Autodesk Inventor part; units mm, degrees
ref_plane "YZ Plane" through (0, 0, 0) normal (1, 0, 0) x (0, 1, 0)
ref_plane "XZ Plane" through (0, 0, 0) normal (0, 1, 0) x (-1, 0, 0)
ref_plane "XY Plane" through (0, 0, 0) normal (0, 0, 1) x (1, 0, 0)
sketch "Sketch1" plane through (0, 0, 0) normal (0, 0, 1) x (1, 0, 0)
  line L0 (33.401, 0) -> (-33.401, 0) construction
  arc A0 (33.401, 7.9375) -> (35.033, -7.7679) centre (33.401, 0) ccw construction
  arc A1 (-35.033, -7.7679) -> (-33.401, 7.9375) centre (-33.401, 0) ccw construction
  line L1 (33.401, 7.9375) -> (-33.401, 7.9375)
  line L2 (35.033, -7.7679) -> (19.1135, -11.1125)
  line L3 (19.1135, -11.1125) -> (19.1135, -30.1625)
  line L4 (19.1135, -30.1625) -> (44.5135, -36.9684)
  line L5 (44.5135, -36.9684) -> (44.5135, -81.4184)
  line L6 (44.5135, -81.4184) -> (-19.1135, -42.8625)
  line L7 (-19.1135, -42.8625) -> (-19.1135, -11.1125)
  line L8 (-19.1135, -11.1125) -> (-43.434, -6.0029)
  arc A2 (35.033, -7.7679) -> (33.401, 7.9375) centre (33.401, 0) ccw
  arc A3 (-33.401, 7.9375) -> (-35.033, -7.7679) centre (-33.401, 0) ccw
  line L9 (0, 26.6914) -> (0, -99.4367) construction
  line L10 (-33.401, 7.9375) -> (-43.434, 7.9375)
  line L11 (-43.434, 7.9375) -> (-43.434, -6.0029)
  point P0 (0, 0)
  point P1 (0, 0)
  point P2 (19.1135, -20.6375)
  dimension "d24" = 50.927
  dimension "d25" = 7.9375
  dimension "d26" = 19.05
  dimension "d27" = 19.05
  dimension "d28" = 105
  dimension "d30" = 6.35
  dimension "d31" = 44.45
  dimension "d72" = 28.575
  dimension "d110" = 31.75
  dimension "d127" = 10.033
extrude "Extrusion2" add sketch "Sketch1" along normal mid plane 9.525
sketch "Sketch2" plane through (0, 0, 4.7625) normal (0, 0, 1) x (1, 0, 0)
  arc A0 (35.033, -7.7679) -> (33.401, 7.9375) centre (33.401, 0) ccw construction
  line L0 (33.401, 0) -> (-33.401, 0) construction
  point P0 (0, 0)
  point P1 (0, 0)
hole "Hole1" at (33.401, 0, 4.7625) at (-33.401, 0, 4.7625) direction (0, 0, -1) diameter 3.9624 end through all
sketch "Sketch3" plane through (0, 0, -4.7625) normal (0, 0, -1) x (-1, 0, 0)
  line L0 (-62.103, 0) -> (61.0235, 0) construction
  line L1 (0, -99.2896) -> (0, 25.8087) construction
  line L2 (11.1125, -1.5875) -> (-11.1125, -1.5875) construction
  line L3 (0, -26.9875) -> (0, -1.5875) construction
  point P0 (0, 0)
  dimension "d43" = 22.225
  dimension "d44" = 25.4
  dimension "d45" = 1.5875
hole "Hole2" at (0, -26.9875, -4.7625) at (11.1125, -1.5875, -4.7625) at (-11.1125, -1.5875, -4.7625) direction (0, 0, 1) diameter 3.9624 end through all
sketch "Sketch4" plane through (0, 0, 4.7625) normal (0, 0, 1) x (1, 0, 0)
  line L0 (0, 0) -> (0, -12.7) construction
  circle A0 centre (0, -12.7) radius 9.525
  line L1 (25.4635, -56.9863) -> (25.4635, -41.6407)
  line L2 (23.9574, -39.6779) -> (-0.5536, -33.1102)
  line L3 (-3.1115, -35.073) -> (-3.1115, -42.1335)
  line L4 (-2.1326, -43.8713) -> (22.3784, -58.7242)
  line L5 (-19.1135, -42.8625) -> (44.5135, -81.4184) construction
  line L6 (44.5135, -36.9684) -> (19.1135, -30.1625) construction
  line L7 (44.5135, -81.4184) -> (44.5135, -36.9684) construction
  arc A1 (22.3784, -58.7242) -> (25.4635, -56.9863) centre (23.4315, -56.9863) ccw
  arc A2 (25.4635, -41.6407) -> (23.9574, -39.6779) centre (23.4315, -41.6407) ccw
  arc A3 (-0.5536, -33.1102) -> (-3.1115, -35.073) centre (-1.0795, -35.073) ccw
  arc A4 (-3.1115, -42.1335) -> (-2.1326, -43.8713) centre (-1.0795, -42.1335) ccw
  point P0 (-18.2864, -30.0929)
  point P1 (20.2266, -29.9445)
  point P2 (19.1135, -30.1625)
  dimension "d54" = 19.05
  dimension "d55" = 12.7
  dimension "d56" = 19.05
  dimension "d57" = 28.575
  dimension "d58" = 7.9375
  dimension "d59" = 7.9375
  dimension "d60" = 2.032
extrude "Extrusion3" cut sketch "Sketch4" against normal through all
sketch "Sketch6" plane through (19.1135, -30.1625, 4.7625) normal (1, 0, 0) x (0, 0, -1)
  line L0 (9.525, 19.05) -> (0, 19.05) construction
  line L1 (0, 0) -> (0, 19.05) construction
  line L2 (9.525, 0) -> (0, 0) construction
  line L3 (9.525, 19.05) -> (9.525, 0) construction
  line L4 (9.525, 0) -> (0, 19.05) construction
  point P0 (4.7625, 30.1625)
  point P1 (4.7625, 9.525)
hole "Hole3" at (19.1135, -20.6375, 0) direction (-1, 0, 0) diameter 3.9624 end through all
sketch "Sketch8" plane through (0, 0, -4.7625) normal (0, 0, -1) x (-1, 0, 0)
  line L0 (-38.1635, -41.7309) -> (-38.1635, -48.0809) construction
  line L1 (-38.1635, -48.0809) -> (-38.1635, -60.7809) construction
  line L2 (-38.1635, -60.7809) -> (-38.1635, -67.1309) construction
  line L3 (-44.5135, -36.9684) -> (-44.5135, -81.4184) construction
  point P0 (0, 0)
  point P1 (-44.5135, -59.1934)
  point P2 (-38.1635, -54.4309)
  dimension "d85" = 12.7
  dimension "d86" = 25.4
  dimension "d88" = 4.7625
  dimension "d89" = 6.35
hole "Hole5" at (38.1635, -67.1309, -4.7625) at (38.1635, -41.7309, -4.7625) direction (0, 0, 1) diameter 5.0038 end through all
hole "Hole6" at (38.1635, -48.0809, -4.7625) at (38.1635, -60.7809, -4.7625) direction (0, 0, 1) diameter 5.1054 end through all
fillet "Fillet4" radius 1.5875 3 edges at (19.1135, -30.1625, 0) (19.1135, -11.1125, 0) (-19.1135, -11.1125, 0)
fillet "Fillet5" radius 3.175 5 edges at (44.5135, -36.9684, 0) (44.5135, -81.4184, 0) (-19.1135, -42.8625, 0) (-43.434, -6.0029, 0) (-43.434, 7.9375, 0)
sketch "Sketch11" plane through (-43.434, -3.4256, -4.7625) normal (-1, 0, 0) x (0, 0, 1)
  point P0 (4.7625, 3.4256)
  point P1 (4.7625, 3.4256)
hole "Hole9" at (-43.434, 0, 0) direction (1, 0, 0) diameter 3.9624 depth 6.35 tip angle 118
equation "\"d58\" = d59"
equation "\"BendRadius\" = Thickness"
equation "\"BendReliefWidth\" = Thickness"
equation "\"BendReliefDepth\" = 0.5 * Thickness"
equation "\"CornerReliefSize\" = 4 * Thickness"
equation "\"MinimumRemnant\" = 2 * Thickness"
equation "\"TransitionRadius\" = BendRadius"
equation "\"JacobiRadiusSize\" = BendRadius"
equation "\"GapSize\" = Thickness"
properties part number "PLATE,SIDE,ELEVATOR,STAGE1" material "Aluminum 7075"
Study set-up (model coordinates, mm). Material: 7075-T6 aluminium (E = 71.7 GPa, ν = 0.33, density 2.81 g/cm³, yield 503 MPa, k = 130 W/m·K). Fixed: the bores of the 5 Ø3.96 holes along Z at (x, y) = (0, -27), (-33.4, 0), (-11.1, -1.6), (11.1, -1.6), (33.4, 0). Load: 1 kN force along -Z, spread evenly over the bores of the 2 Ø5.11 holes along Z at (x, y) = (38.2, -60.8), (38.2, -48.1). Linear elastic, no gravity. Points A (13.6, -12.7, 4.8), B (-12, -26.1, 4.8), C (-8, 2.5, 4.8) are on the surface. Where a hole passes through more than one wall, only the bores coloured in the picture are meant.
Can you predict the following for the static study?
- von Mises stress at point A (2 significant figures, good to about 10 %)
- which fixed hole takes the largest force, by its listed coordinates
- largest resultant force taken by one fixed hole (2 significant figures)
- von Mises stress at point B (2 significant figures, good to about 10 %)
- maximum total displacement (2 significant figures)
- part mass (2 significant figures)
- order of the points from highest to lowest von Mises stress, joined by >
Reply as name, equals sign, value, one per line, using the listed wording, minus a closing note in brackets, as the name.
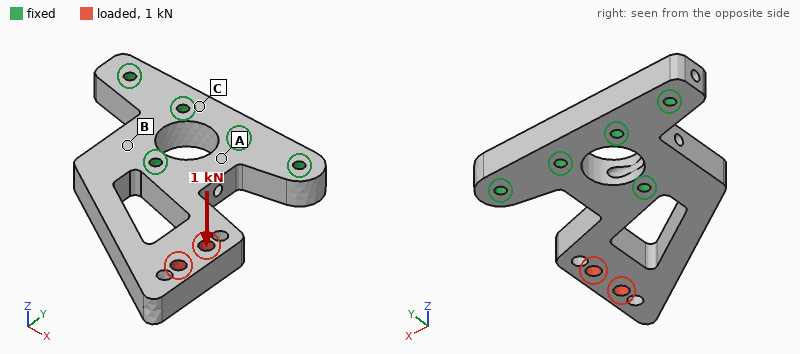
von Mises stress at point A = 61 MPa
which fixed hole takes the largest force, by its listed coordinates = (0, -27)
largest resultant force taken by one fixed hole = 1.4 kN
von Mises stress at point B = 38 MPa
maximum total displacement = 0.65 mm
part mass = 86 g
order of the points from highest to lowest von Mises stress, joined by > = A > B > C
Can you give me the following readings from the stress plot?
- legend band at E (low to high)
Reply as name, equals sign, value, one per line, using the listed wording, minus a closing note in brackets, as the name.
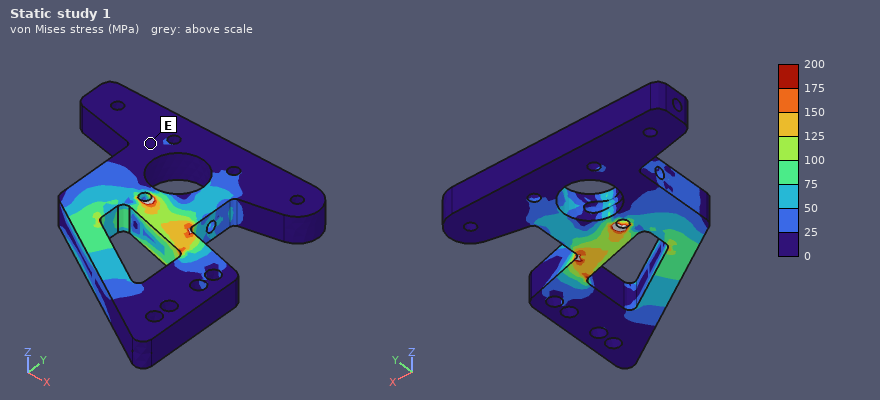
legend band at E = 0 to 25 MPa
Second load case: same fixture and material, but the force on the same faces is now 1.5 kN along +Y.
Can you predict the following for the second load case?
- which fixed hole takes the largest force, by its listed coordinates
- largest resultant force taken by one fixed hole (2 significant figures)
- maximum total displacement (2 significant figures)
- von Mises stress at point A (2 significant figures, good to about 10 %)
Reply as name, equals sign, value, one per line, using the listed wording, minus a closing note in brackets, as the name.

which fixed hole takes the largest force, by its listed coordinates = (11.1, -1.6)
largest resultant force taken by one fixed hole = 1.8 kN
maximum total displacement = 0.11 mm
von Mises stress at point A = 25 MPa
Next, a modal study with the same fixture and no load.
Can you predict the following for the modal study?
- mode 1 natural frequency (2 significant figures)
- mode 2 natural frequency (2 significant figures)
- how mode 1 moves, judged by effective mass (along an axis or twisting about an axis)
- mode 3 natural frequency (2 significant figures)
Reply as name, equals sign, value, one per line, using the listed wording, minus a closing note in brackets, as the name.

mode 1 natural frequency = 1700 Hz
mode 2 natural frequency = 4100 Hz
how mode 1 moves, judged by effective mass = along Z
mode 3 natural frequency = 5200 Hz
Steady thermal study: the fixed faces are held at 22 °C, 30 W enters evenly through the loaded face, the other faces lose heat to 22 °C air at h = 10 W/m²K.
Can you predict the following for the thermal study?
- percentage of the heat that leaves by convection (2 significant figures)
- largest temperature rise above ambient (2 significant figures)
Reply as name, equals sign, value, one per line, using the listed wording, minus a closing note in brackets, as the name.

percentage of the heat that leaves by convection = 7.0 %
largest temperature rise above ambient = 61 K
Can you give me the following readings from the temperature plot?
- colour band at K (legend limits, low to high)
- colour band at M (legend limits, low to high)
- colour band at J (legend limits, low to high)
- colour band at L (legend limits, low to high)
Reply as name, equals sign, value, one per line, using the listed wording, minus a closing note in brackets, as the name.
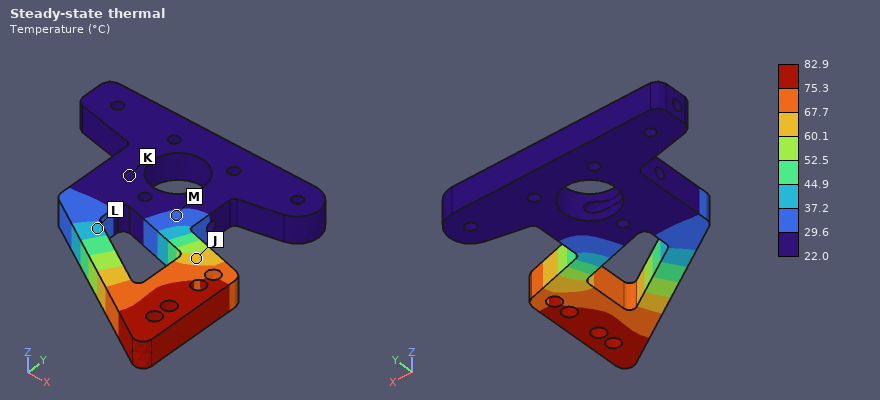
colour band at K = 22.0 to 29.6 °C
colour band at M = 29.6 to 37.2 °C
colour band at J = 60.1 to 67.7 °C
colour band at L = 37.2 to 44.9 °C
